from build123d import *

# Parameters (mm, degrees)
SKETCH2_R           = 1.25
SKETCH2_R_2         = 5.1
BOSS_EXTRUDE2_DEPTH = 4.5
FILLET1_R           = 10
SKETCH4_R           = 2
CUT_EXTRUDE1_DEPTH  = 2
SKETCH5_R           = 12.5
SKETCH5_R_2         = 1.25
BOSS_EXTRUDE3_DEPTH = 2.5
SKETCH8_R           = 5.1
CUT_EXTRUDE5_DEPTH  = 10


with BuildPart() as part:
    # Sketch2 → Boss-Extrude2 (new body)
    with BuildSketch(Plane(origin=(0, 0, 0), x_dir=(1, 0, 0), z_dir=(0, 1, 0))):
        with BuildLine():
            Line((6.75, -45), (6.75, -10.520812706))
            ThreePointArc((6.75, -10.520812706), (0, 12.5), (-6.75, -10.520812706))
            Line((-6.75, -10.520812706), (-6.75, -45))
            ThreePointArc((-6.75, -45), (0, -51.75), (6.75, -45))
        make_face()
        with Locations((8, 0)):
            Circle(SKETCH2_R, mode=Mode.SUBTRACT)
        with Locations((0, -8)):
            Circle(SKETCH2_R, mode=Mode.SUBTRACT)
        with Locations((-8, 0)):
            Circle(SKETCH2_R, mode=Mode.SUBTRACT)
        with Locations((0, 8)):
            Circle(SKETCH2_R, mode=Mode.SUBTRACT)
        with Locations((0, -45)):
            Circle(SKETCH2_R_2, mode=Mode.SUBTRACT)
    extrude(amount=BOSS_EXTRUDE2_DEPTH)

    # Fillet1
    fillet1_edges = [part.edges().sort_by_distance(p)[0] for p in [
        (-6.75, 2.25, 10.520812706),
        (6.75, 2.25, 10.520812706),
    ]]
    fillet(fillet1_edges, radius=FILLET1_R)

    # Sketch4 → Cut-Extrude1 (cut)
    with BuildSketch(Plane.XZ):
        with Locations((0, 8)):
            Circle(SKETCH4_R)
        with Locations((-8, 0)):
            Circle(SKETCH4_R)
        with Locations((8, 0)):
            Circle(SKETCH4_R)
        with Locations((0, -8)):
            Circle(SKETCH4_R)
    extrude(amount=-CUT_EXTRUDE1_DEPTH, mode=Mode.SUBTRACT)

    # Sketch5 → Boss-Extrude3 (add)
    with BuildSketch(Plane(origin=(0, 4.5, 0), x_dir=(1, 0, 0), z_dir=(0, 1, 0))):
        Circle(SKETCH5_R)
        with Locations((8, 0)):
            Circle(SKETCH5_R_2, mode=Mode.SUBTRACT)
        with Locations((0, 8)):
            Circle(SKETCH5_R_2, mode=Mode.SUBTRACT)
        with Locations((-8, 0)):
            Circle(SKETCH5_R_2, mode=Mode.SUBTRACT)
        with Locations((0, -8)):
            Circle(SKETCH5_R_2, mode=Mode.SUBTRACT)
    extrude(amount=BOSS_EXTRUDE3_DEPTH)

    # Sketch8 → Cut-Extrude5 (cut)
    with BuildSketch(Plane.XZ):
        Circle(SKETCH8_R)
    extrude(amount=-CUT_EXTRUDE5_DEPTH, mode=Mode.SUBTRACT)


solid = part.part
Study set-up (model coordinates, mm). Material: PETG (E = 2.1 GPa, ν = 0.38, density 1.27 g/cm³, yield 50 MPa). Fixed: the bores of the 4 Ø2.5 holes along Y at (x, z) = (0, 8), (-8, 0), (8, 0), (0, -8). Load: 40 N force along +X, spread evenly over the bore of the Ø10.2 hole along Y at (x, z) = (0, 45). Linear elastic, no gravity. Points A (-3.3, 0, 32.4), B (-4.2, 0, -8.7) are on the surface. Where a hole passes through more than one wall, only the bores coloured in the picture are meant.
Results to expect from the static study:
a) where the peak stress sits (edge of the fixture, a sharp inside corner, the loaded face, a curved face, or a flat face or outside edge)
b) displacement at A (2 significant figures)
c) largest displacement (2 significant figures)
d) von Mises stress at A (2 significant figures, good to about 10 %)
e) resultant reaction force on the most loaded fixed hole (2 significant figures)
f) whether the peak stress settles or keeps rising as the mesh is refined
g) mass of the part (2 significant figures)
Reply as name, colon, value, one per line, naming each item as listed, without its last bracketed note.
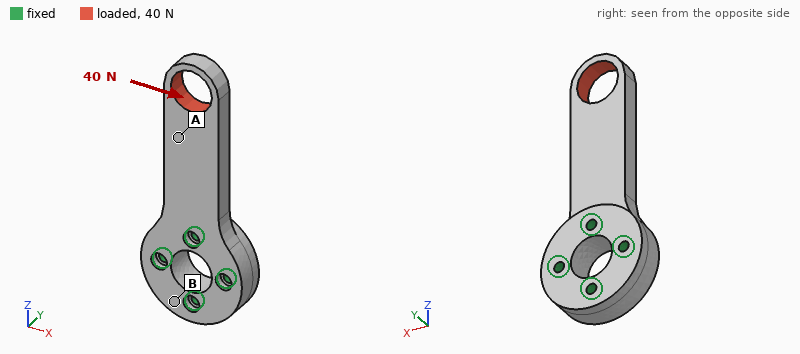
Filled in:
where the peak stress sits: edge of the fixture
displacement at A: 0.21 mm
largest displacement: 0.61 mm
von Mises stress at A: 2.0 MPa
resultant reaction force on the most loaded fixed hole: 88 N
whether the peak stress settles or keeps rising as the mesh is refined: keeps rising
mass of the part: 5.9 g
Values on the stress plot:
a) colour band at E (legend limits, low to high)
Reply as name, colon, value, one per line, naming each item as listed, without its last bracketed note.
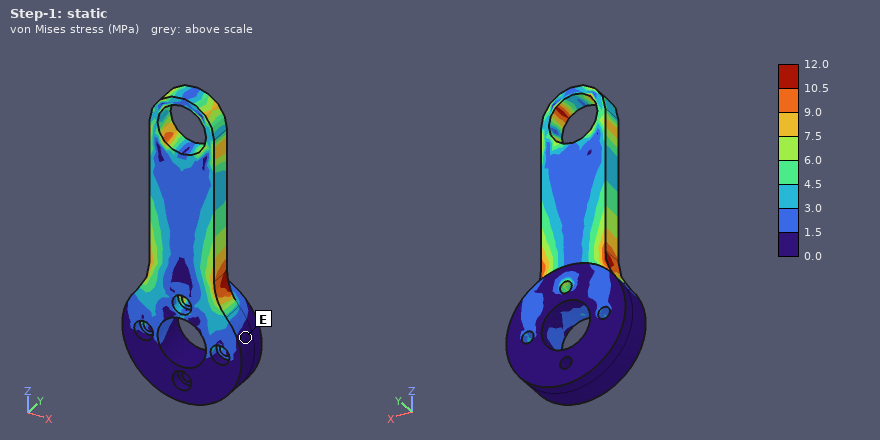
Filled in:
colour band at E: 0.0 to 1.5 MPa
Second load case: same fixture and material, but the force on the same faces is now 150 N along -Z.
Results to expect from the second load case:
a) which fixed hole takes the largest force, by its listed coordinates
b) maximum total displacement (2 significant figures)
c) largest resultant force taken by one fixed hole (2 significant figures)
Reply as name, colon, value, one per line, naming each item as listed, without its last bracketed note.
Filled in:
which fixed hole takes the largest force, by its listed coordinates: (0, 8)
maximum total displacement: 0.16 mm
largest resultant force taken by one fixed hole: 83 N
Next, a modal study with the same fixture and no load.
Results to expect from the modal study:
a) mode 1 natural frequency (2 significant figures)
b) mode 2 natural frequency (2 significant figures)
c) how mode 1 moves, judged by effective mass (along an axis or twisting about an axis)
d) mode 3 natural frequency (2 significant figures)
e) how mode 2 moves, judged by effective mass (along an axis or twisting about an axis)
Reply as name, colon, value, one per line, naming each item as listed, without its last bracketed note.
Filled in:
mode 1 natural frequency: 710 Hz
mode 2 natural frequency: 1800 Hz
how mode 1 moves, judged by effective mass: along Y
mode 3 natural frequency: 3000 Hz
how mode 2 moves, judged by effective mass: along X
